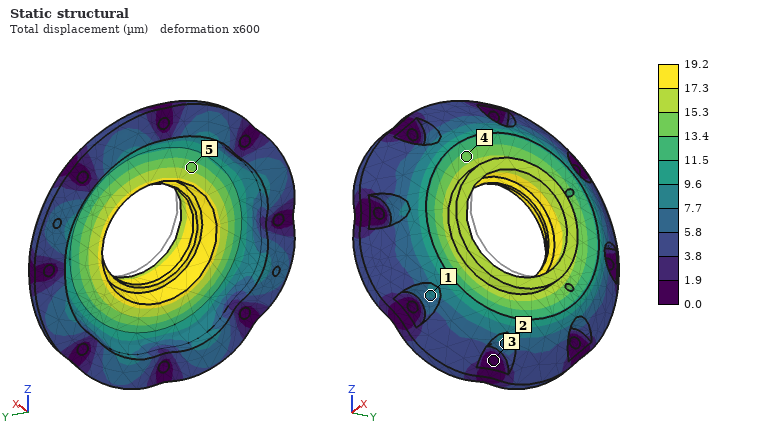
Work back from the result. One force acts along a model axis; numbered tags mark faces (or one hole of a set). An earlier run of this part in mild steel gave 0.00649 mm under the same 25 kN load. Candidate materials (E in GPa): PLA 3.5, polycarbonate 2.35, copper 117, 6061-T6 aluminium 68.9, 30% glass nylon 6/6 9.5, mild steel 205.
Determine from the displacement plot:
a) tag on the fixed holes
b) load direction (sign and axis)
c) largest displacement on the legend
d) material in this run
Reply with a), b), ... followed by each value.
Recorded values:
a) 3
b) -X
c) 19.2 µm
d) 6061-T6 aluminium
